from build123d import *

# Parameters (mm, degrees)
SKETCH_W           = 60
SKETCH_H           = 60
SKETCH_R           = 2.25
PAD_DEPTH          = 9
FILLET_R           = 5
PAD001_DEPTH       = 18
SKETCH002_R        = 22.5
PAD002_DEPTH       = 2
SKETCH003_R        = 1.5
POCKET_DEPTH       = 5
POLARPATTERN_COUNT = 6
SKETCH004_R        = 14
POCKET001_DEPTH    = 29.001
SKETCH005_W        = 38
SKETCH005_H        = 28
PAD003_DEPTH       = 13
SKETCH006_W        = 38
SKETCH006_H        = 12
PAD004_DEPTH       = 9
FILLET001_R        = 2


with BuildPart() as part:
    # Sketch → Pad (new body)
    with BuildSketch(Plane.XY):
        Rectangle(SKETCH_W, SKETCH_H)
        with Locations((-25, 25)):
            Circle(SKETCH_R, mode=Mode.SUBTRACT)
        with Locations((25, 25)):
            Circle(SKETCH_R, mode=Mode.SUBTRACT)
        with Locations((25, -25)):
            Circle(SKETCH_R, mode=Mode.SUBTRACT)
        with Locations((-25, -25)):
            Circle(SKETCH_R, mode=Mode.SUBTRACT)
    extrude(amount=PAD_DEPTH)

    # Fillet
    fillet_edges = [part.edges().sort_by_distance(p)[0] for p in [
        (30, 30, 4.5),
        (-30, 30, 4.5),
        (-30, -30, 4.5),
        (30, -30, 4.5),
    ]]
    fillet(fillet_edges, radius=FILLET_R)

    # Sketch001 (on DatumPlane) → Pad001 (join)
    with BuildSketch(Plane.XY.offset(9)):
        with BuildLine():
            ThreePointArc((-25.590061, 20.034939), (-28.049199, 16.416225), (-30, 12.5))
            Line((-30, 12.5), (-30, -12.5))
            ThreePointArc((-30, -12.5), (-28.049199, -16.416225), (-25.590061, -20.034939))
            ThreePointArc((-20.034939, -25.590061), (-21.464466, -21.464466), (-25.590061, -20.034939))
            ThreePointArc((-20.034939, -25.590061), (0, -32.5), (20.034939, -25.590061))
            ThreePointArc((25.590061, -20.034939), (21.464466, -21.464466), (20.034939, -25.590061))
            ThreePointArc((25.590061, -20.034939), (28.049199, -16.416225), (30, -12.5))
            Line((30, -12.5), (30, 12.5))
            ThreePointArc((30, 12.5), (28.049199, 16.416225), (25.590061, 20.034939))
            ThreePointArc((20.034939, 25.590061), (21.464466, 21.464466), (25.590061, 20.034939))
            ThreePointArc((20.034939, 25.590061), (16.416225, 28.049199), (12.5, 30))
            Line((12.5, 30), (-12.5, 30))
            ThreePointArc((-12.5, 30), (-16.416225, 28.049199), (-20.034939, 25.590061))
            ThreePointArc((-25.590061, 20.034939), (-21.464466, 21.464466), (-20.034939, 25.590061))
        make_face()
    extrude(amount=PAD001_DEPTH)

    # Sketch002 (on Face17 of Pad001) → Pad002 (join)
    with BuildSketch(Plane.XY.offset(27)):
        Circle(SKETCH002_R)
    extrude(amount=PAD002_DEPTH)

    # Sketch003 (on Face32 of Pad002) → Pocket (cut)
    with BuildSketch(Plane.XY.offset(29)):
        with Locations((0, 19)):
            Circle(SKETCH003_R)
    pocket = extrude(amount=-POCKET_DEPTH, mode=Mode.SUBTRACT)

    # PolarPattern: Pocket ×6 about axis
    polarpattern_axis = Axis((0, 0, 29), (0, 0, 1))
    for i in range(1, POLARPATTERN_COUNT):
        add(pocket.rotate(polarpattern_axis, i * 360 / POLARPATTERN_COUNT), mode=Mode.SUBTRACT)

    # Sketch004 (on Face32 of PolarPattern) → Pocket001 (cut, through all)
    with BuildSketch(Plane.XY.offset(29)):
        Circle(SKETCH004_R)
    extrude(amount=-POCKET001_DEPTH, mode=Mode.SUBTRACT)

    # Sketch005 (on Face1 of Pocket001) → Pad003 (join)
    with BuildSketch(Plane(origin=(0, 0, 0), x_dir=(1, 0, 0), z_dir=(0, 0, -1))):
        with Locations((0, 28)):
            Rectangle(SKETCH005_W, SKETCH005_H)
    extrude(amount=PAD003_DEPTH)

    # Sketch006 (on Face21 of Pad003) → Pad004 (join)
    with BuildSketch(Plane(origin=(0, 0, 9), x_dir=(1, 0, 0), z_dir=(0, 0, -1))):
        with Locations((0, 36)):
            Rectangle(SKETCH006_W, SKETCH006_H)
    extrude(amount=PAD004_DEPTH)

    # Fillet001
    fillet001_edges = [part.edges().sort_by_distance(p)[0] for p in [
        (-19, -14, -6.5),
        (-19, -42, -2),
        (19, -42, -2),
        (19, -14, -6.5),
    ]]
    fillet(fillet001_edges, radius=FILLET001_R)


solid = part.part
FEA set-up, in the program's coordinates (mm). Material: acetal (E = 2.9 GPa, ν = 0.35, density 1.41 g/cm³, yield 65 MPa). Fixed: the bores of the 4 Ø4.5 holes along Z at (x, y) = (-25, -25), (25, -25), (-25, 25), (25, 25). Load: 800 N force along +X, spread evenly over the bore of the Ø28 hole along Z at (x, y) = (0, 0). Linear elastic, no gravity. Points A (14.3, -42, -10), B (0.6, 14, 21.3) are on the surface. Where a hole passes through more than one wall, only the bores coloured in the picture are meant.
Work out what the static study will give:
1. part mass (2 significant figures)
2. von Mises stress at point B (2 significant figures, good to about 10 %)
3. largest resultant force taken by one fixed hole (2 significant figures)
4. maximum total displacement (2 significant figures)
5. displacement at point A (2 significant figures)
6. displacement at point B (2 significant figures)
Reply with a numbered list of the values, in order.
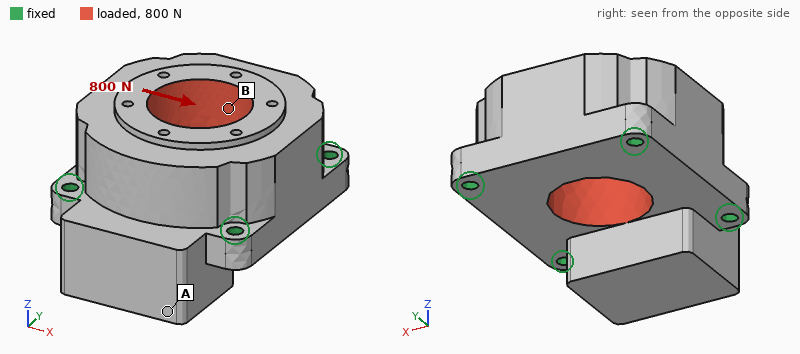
1. 130 g
2. 0.78 MPa
3. 230 N
4. 19 µm
5. 3.1 µm
6. 14 µm
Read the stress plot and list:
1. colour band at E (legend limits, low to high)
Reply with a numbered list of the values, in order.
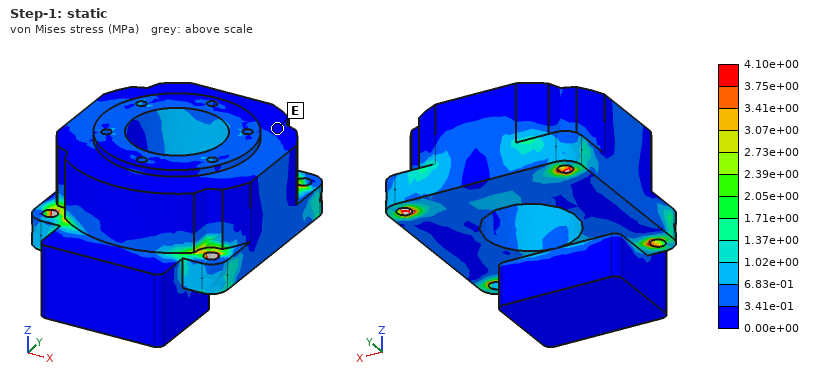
1. 0.00e+00 to 3.41e-01 MPa
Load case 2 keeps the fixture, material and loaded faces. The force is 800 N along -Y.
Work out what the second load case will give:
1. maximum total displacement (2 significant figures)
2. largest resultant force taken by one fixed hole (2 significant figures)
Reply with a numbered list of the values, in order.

1. 20 µm
2. 230 N
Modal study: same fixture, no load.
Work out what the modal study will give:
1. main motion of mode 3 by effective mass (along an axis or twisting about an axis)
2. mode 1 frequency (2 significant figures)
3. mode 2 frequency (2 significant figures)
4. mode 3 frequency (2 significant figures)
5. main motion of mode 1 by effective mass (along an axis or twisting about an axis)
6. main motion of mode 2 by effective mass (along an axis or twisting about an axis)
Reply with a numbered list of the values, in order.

1. along X
2. 2800 Hz
3. 3500 Hz
4. 3900 Hz
5. along Z
6. along Z
